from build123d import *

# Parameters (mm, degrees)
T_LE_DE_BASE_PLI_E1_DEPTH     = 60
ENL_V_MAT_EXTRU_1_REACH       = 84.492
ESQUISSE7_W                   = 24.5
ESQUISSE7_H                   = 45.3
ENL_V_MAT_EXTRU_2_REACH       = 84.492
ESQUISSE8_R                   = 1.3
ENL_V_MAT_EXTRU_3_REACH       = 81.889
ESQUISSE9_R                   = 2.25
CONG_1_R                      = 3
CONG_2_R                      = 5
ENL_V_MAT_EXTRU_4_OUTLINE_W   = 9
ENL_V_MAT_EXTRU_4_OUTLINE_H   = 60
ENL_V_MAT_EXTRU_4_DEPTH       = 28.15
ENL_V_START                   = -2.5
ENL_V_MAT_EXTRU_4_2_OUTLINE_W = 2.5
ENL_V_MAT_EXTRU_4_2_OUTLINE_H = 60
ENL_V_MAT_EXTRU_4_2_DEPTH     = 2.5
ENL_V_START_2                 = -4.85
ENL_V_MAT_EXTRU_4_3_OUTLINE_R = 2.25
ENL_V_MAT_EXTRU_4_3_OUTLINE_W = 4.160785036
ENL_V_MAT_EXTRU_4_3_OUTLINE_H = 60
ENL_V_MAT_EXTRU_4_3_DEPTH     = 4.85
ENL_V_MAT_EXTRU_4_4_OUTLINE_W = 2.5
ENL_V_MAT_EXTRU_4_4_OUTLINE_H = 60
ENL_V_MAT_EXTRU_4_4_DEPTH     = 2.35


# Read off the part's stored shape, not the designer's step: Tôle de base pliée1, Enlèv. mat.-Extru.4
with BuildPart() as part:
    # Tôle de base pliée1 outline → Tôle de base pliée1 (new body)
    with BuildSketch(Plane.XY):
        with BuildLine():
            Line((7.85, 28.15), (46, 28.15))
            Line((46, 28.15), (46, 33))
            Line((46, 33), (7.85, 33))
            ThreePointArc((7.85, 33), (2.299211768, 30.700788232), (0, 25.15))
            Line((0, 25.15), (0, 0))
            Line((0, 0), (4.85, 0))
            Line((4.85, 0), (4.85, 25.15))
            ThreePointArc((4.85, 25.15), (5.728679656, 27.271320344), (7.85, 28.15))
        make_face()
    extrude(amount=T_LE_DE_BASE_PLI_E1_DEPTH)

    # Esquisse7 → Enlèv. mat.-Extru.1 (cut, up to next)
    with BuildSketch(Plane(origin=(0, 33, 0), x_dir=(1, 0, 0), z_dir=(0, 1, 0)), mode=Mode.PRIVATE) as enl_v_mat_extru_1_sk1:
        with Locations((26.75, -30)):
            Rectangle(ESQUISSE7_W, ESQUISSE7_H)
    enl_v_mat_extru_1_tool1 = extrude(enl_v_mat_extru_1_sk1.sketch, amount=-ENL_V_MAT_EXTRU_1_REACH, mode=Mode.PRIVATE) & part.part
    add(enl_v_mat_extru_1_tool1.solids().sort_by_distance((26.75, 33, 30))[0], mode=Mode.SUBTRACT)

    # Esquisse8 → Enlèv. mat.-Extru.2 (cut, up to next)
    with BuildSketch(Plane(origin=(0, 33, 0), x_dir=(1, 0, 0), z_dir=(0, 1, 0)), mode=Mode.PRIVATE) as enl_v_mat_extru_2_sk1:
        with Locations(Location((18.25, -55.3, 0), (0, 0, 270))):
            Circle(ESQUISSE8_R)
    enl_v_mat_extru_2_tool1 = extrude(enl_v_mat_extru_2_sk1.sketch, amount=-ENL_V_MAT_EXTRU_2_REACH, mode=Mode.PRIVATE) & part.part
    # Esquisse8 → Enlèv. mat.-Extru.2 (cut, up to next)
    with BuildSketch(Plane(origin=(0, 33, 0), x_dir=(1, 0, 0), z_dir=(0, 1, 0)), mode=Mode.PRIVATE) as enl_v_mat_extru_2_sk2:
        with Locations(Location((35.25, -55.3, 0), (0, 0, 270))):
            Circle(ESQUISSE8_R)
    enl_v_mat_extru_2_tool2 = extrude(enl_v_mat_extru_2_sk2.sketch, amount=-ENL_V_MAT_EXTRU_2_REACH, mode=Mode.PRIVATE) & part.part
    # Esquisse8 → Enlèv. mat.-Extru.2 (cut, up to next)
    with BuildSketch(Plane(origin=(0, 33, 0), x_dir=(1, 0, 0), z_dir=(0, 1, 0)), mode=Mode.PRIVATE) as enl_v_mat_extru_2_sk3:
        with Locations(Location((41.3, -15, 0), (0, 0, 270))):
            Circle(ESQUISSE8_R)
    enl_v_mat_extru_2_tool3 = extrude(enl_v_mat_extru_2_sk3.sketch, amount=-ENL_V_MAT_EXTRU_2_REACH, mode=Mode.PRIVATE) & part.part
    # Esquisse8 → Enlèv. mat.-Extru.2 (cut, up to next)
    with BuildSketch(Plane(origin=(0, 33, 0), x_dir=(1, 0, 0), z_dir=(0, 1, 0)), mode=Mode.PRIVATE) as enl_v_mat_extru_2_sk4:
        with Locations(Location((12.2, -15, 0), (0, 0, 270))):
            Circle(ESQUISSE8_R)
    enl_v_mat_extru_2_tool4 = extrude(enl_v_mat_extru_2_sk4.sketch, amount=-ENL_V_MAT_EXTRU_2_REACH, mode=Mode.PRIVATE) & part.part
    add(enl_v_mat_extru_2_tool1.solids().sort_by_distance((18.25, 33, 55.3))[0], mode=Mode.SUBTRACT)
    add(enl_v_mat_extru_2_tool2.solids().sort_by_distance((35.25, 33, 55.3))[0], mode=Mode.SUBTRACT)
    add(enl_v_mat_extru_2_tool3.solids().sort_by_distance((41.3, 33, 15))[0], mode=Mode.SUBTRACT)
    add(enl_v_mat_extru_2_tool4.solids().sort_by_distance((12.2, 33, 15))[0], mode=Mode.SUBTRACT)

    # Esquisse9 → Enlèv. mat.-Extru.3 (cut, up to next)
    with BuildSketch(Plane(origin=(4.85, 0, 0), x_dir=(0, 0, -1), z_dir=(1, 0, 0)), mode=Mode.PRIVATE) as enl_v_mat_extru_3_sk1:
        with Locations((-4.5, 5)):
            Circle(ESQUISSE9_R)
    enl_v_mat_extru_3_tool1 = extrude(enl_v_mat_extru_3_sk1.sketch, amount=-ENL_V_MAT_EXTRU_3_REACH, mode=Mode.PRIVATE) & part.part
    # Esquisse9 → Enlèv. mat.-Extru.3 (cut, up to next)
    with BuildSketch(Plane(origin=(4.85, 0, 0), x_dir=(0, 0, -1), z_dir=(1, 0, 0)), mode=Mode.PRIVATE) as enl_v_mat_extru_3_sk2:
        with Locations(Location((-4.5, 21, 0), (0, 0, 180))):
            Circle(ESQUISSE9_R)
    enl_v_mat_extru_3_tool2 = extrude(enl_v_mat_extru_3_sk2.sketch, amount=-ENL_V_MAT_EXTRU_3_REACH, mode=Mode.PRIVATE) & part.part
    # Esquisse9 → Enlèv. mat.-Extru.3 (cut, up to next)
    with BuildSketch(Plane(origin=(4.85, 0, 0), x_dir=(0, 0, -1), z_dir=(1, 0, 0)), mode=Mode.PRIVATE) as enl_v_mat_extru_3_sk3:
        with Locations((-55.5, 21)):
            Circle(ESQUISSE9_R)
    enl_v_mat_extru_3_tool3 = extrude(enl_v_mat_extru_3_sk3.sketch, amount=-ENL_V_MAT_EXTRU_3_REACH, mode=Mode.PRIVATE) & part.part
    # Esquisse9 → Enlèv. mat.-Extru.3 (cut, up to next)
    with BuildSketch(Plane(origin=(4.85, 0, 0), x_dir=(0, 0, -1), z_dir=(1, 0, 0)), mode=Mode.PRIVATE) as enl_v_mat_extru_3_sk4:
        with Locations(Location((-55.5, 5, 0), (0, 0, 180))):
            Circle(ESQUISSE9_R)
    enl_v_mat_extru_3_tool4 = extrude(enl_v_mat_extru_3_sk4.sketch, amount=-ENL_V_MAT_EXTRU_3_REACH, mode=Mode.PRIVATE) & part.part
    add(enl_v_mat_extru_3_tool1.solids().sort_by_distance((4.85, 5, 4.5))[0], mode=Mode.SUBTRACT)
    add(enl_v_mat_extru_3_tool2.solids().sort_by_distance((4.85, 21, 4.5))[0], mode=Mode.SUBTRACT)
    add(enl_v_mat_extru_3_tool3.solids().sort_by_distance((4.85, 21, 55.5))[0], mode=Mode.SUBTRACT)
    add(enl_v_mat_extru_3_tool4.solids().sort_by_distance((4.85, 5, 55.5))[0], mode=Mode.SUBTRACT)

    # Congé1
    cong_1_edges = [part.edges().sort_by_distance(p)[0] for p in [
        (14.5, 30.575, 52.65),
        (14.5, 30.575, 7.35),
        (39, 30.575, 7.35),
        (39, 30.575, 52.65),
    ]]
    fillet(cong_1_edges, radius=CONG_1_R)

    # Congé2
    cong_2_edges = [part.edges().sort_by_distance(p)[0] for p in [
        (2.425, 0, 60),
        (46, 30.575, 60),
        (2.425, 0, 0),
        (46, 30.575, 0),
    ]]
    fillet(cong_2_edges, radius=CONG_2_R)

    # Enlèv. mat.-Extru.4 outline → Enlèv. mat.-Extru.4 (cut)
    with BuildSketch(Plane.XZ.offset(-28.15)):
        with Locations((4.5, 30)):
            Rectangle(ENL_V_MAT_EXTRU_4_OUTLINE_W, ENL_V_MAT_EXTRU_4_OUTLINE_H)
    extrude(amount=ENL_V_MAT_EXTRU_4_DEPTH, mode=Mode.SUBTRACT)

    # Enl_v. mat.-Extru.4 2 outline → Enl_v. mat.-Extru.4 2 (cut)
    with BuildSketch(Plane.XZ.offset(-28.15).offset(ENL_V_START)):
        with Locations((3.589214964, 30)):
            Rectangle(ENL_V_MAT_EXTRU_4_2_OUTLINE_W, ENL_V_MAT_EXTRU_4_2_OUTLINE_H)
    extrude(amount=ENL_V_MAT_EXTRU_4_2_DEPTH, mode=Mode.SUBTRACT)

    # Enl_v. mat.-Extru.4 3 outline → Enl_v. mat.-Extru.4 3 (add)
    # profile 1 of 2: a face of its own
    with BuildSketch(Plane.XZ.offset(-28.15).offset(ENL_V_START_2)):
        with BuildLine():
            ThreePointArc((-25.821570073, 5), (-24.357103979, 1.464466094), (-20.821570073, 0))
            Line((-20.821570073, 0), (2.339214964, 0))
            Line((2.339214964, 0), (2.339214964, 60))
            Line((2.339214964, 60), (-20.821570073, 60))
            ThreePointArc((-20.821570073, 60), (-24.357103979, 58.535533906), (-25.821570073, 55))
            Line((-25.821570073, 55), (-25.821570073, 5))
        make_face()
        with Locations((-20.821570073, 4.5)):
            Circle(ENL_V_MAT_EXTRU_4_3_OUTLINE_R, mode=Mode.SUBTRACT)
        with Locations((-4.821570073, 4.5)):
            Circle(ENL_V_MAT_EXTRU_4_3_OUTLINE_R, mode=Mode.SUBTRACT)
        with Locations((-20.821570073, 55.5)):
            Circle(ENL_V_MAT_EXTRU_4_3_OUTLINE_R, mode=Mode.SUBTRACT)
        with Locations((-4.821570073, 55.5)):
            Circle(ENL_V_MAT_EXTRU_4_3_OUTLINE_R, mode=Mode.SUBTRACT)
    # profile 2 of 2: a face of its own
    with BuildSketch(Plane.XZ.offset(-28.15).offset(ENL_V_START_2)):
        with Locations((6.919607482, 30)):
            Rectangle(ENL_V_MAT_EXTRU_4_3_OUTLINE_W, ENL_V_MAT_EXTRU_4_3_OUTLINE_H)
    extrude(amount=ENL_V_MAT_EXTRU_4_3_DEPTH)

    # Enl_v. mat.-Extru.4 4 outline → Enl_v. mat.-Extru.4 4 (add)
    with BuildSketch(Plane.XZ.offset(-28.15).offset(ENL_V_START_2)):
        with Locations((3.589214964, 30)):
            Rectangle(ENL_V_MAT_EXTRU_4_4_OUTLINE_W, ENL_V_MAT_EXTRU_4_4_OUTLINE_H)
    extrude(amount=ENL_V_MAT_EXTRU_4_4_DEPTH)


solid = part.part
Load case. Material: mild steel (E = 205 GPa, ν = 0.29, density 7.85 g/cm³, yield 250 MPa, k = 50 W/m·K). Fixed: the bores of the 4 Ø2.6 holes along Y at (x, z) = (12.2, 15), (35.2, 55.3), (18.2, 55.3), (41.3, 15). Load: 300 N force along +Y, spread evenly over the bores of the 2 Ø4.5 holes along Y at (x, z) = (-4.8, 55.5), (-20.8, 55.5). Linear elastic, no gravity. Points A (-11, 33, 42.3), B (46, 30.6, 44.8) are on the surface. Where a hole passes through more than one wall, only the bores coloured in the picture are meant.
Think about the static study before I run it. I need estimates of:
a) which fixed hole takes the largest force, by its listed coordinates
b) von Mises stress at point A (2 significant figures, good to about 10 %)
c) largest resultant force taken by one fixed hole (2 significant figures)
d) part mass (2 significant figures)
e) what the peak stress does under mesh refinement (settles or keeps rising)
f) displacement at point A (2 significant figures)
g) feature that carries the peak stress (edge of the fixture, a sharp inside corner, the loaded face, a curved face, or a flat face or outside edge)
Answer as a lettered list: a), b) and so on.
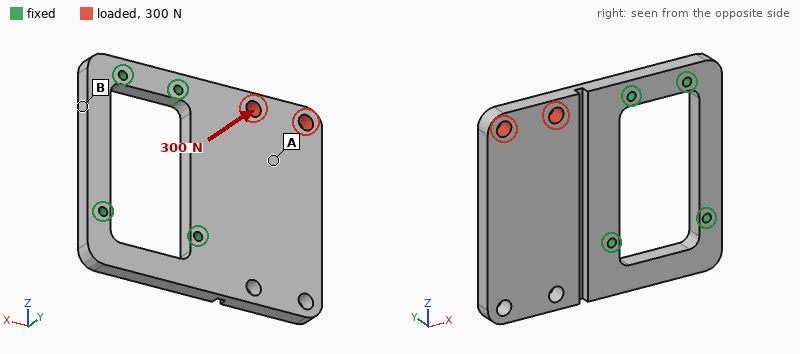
a) (18.2, 55.3)
b) 25 MPa
c) 300 N
d) 120 g
e) keeps rising
f) 0.072 mm
g) edge of the fixture
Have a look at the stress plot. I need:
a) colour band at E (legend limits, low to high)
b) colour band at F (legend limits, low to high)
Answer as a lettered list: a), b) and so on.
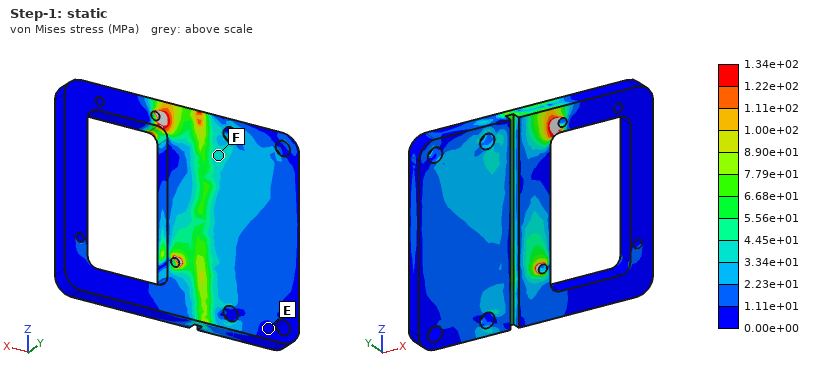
a) 0.00e+00 to 1.11e+01 MPa
b) 3.34e+01 to 4.45e+01 MPa
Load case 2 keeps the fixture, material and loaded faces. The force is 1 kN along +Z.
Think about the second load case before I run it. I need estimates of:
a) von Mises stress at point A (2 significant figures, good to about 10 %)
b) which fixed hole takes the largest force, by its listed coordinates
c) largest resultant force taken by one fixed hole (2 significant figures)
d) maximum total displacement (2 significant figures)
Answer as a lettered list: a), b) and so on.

a) 8.6 MPa
b) (12.2, 15)
c) 890 N
d) 5.8 µm
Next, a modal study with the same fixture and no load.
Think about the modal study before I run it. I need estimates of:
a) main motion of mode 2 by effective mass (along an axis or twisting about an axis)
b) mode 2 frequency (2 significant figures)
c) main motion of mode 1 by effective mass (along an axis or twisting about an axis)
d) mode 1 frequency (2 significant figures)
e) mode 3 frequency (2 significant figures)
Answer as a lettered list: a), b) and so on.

a) twisting about X
b) 3700 Hz
c) along Y
d) 1400 Hz
e) 8800 Hz
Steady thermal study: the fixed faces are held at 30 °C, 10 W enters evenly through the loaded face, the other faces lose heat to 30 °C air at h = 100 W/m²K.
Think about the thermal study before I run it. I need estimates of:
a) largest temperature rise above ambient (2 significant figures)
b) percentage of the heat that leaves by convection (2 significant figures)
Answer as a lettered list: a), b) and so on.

a) 36 K
b) 63 %
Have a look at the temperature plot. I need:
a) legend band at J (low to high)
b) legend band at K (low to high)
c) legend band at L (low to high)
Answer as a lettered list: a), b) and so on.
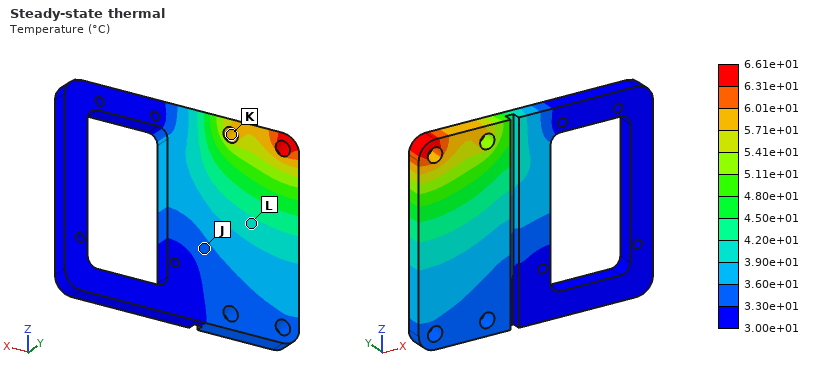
a) 3.30e+01 to 3.60e+01 °C
b) 5.71e+01 to 6.01e+01 °C
c) 3.90e+01 to 4.20e+01 °C
